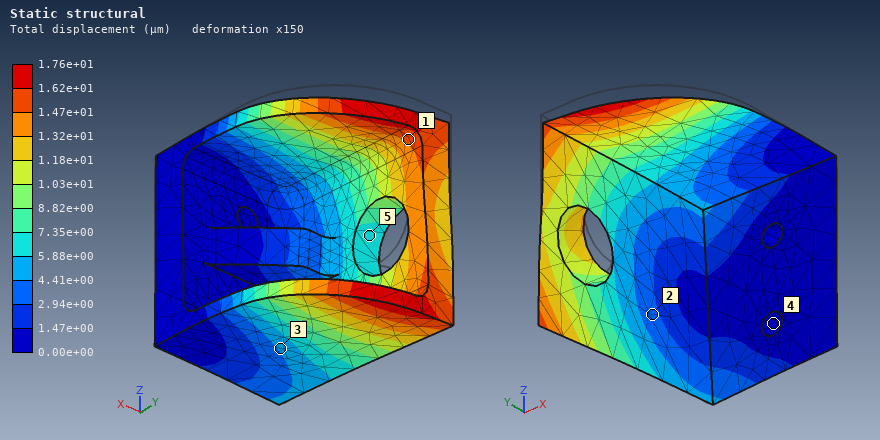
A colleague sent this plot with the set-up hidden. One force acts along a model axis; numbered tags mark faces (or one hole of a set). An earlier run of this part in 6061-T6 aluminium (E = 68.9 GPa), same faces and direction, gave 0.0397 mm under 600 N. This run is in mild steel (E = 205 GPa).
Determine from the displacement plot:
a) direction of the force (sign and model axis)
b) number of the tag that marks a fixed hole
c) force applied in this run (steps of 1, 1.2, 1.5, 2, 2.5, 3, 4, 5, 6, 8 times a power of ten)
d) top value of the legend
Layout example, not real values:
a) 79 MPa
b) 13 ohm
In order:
a) -Z
b) 4
c) 800 N
d) 1.76e+01 µm
